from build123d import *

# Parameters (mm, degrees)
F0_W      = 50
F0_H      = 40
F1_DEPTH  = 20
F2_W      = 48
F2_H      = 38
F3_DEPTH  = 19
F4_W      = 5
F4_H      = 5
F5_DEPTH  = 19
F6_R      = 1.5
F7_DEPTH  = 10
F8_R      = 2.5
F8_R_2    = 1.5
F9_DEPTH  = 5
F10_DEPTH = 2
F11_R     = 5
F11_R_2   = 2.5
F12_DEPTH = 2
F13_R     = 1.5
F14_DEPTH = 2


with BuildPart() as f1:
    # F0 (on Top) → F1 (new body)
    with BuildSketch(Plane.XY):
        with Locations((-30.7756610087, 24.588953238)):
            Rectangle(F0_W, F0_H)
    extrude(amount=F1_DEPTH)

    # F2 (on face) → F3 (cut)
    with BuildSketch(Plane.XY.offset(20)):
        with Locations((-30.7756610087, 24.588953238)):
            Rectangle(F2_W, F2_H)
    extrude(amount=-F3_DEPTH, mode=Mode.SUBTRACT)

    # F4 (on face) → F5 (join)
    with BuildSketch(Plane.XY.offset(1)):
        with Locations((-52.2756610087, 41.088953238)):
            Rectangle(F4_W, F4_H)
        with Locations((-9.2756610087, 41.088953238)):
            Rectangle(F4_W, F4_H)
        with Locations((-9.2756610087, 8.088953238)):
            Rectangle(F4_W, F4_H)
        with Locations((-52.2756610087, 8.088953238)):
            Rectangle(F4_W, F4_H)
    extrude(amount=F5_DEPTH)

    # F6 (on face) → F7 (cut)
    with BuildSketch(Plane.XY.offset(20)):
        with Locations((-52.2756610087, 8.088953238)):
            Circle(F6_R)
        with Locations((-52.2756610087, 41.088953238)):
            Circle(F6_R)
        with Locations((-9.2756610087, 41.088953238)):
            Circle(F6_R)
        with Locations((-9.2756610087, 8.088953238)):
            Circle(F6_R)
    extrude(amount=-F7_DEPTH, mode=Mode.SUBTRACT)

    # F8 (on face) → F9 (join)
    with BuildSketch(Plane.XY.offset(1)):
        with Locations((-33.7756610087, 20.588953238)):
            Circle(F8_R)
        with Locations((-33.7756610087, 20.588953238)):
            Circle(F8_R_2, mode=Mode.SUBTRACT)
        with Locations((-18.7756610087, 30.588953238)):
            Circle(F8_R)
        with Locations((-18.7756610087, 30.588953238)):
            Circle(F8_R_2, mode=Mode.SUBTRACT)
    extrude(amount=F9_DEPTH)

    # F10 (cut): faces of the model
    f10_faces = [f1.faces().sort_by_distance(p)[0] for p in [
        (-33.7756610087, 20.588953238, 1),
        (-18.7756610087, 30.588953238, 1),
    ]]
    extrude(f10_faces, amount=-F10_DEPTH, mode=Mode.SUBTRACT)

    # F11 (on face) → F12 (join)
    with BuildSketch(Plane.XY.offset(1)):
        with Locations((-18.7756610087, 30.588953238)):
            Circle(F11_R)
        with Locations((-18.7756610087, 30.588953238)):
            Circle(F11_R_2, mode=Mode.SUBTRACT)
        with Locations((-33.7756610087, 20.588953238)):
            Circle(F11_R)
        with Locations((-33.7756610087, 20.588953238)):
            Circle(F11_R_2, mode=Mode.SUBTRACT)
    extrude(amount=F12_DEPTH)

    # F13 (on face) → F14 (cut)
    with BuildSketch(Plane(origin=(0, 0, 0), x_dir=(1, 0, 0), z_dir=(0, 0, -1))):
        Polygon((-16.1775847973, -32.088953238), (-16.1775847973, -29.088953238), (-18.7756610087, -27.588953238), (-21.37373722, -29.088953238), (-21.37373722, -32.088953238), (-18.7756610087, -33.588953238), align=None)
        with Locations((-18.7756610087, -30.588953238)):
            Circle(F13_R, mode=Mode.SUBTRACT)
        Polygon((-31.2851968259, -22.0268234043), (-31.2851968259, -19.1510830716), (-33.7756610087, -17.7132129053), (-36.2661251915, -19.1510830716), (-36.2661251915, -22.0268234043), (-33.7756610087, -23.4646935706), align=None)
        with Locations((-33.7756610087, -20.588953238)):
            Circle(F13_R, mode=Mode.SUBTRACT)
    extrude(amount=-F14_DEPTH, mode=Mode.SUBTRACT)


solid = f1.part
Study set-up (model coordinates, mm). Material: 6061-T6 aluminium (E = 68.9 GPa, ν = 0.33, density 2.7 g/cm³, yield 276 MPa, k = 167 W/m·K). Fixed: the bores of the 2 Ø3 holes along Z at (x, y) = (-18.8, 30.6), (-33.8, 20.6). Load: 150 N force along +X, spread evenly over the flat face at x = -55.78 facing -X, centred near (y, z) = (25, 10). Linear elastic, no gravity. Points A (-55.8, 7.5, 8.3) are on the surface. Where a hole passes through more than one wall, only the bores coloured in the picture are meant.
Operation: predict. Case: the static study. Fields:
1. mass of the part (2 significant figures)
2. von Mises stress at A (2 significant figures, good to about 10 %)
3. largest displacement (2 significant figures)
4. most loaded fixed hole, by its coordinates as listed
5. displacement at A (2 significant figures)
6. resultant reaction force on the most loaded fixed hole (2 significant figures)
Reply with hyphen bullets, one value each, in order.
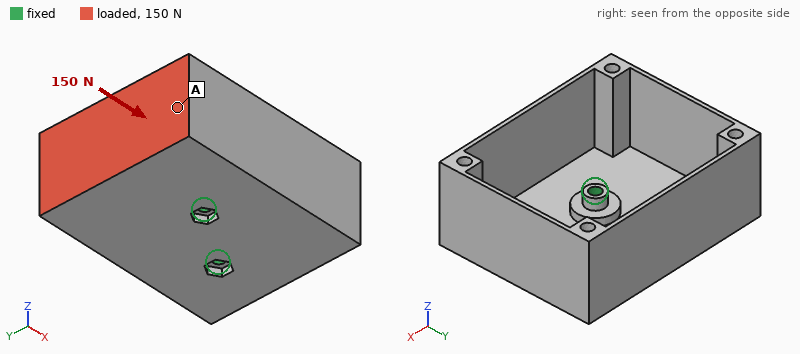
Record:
- 20 g
- 10 MPa
- 0.22 mm
- (-33.8, 20.6)
- 0.11 mm
- 89 N
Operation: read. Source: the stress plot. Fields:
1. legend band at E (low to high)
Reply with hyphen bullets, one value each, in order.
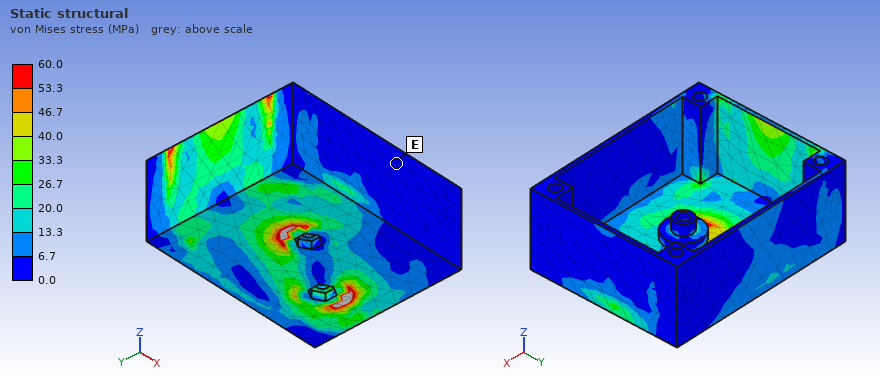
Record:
- 0.0 to 6.7 MPa
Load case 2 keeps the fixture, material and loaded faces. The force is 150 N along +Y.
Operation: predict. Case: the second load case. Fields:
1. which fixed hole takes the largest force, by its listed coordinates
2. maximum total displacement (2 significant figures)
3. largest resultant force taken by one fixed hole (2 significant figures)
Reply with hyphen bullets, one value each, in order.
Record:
- (-33.8, 20.6)
- 0.51 mm
- 270 N
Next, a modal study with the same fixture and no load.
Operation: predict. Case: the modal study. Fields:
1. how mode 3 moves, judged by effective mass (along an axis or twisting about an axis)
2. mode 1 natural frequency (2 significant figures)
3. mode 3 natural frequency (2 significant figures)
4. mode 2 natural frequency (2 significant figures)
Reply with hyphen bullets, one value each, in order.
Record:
- along Z
- 810 Hz
- 1300 Hz
- 1000 Hz
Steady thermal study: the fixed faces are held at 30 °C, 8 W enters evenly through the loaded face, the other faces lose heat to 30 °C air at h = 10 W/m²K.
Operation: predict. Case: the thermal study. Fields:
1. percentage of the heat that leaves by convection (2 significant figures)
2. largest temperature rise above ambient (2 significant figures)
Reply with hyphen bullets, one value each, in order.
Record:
- 13 %
- 24 K
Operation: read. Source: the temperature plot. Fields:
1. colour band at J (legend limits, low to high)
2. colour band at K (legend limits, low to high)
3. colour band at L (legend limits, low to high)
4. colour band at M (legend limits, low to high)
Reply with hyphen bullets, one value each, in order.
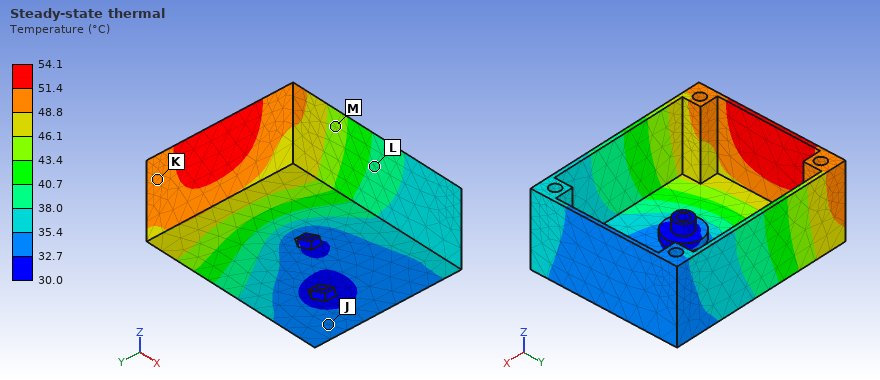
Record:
- 32.7 to 35.4 °C
- 48.8 to 51.4 °C
- 38.0 to 40.7 °C
- 43.4 to 46.1 °C
